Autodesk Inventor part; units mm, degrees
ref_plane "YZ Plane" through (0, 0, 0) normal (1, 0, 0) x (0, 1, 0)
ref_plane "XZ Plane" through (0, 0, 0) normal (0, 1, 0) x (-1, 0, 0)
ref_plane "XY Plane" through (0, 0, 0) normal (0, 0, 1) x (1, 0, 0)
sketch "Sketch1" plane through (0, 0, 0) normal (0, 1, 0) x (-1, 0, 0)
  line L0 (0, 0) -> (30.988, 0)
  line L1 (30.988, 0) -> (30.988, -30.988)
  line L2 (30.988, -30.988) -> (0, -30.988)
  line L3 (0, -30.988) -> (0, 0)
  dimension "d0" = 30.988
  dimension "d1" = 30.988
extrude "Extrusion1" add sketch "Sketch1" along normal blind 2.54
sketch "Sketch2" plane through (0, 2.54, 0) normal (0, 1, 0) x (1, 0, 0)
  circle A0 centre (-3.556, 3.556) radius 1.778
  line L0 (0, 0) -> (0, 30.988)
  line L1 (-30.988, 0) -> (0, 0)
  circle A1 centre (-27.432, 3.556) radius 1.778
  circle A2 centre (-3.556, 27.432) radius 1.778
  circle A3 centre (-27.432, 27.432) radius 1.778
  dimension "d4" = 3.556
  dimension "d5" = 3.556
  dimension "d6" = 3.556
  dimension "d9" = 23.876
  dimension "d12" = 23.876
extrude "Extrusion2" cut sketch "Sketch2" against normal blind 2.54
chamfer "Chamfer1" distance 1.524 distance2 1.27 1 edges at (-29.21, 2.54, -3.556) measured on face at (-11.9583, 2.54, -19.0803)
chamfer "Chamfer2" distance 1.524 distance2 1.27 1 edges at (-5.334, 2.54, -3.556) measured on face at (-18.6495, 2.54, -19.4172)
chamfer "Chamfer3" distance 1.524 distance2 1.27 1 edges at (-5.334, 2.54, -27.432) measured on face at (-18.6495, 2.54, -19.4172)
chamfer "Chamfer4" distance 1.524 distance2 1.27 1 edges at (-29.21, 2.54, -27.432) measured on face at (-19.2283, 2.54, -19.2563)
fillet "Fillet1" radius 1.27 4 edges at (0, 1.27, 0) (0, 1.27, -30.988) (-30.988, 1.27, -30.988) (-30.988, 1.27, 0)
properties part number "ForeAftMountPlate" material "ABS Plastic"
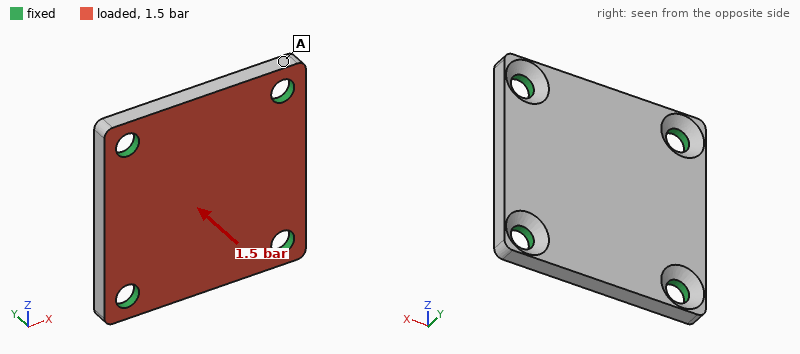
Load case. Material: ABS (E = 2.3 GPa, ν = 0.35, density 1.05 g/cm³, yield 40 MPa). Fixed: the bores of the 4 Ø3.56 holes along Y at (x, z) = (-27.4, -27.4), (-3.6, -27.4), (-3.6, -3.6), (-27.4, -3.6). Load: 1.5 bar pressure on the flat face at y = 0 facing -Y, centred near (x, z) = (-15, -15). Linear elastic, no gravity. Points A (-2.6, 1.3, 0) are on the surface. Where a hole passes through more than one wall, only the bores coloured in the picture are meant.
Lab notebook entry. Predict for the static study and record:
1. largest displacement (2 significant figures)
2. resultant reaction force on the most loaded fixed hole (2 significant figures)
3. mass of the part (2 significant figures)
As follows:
0.11 mm
42 N
2.4 g
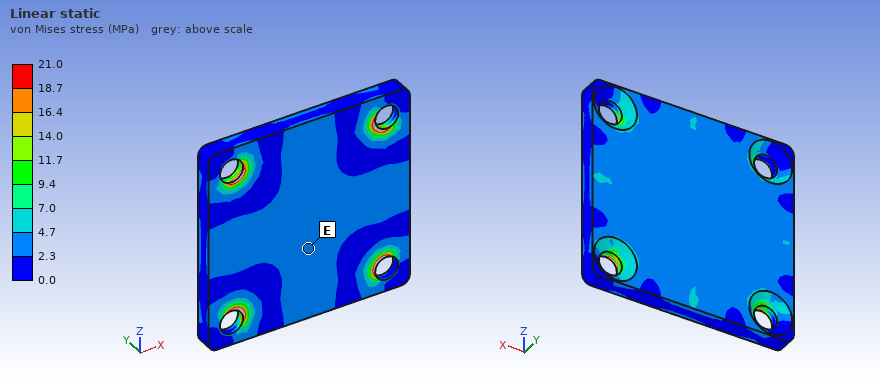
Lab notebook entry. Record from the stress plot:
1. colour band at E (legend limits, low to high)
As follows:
2.3 to 4.7 MPa
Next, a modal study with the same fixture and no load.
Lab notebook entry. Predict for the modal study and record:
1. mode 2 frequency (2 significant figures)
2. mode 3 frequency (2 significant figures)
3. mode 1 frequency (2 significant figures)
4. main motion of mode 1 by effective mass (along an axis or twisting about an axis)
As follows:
6800 Hz
6800 Hz
4400 Hz
along Y
